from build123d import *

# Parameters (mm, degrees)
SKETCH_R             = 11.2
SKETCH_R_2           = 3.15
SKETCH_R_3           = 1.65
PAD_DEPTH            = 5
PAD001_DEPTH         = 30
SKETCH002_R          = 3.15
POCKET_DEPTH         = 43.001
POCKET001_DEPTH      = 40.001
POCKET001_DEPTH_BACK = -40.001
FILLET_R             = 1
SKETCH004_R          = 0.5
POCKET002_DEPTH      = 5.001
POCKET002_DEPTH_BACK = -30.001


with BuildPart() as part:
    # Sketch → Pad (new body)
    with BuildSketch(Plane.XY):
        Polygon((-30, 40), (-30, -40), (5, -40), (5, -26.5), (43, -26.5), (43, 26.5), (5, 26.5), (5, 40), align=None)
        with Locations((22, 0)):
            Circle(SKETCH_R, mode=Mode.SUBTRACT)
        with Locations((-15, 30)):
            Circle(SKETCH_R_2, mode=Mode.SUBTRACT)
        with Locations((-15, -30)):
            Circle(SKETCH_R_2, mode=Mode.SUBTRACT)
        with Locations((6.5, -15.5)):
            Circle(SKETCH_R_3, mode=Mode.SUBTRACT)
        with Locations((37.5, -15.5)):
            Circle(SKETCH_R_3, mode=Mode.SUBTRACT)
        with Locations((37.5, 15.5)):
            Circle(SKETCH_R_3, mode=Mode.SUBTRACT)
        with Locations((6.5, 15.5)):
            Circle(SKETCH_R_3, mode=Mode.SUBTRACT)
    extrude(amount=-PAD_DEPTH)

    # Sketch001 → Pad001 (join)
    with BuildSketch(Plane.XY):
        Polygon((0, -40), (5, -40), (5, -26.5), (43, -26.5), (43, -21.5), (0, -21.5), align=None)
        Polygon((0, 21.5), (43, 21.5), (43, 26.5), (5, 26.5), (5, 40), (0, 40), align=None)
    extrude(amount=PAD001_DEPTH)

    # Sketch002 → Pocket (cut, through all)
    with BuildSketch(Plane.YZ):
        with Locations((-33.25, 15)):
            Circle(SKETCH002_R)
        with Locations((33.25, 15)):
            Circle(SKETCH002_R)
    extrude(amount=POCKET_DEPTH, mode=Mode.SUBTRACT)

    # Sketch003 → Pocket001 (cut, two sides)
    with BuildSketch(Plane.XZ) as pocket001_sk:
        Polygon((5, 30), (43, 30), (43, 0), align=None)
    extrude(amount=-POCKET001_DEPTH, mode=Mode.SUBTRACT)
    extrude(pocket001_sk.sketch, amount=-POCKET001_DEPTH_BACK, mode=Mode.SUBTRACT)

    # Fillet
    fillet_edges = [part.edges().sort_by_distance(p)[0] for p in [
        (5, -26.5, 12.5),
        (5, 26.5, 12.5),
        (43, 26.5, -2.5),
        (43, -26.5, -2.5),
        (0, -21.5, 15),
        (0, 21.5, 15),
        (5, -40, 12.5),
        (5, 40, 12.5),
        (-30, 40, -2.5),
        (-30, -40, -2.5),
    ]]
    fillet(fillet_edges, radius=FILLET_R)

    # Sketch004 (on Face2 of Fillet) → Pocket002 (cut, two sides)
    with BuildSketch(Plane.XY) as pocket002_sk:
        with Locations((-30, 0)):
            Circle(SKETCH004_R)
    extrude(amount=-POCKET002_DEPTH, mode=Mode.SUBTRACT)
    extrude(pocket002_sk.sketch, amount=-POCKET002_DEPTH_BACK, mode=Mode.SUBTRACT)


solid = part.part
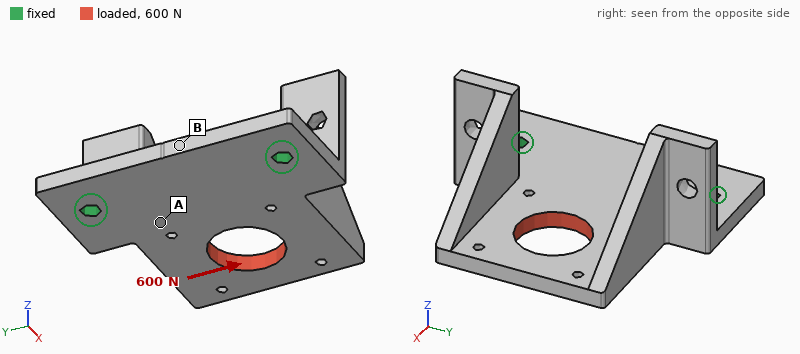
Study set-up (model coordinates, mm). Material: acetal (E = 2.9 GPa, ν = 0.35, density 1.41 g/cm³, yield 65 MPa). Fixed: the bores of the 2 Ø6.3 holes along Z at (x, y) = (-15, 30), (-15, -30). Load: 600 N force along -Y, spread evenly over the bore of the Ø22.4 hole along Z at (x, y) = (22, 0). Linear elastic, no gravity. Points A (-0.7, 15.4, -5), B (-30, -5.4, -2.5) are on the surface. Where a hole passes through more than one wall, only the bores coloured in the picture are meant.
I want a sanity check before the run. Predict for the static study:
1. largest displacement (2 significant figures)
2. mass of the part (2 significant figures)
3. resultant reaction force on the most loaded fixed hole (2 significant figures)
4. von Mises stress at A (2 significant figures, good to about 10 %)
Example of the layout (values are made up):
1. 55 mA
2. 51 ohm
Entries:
1. 0.20 mm
2. 46 g
3. 460 N
4. 3.2 MPa
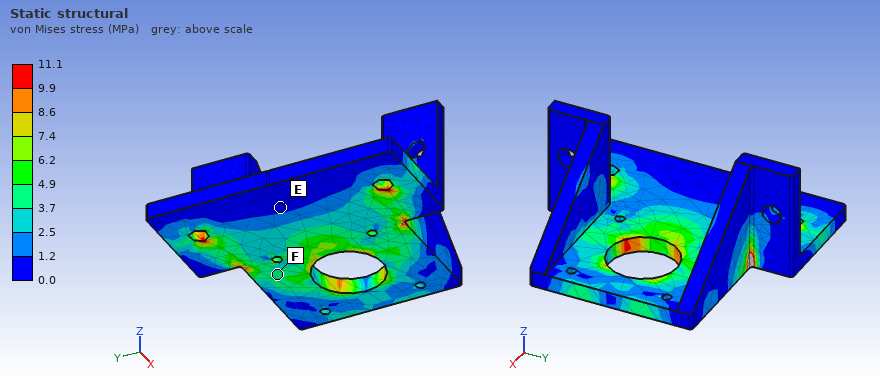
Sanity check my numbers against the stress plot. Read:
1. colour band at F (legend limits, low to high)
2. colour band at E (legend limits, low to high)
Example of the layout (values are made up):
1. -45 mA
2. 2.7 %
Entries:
1. 3.7 to 4.9 MPa
2. 0.0 to 1.2 MPa
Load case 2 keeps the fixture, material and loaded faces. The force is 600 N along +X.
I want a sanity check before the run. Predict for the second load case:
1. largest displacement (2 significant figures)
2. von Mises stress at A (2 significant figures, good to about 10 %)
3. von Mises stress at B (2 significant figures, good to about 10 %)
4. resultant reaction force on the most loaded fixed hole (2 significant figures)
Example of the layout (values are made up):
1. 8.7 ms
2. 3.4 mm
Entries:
1. 93 µm
2. 2.4 MPa
3. 2.0 MPa
4. 320 N
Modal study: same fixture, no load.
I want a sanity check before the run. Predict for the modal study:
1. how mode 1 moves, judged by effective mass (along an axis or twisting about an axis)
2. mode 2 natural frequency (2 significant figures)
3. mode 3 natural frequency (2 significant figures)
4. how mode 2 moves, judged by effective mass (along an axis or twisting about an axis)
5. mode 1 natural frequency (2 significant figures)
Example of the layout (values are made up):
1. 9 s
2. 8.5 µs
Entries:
1. along Z
2. 680 Hz
3. 1000 Hz
4. twisting about X
5. 340 Hz
